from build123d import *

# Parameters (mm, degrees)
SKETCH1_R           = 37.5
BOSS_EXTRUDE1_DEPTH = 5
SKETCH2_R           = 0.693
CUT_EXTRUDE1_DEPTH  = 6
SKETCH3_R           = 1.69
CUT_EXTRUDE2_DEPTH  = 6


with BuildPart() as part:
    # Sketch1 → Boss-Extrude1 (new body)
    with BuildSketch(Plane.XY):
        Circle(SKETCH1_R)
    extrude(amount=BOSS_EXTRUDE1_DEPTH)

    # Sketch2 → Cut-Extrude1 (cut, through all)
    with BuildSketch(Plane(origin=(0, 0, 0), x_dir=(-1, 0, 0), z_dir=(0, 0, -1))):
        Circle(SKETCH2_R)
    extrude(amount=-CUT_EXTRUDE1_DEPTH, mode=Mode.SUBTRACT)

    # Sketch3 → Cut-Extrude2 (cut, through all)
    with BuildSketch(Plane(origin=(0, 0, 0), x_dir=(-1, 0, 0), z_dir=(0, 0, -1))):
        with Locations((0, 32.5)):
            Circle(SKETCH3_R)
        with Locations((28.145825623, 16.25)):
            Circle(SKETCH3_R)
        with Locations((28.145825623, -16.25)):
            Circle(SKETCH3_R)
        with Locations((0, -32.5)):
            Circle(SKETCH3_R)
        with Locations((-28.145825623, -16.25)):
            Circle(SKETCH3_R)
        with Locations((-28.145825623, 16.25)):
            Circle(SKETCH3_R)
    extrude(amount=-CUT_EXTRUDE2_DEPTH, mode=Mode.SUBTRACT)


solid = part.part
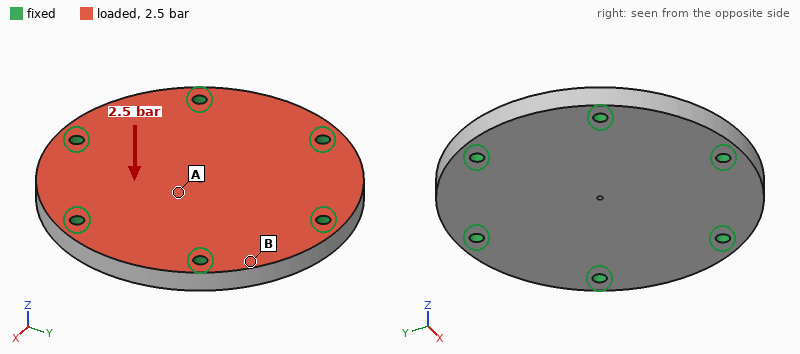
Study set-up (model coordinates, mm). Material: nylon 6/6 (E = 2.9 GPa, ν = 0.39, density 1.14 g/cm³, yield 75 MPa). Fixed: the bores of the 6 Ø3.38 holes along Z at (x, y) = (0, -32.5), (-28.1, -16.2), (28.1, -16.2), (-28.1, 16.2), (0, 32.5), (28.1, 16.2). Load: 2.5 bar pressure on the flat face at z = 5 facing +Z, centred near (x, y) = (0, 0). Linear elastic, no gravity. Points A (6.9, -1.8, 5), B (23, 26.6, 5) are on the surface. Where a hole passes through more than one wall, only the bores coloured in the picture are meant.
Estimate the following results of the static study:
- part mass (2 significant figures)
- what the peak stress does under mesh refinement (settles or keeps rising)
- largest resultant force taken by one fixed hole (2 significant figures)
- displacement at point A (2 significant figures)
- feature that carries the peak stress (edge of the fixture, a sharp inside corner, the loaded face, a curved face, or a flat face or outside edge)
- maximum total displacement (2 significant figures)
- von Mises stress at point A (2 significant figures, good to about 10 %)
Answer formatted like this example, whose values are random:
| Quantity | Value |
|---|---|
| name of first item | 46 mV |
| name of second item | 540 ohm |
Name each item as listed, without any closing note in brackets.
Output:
| Quantity | Value |
|---|---|
| part mass | 25 g |
| what the peak stress does under mesh refinement | keeps rising |
| largest resultant force taken by one fixed hole | 180 N |
| displacement at point A | 0.18 mm |
| feature that carries the peak stress | edge of the fixture |
| maximum total displacement | 0.20 mm |
| von Mises stress at point A | 5.7 MPa |
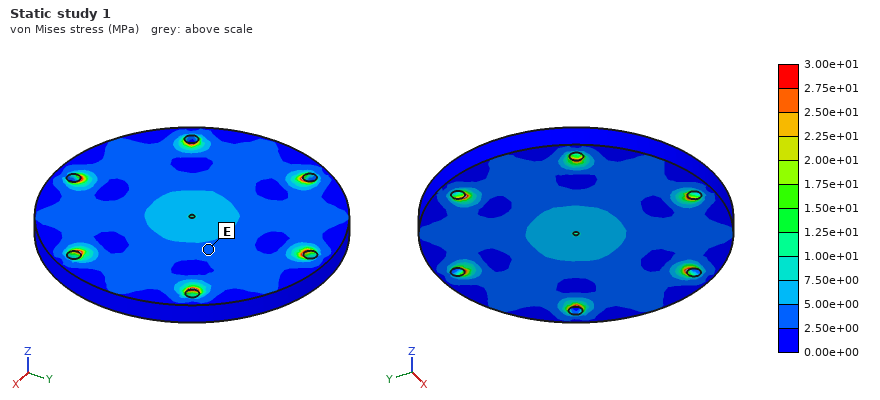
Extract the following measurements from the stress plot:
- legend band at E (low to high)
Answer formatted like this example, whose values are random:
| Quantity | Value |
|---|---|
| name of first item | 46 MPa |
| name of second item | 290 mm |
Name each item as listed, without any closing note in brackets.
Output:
| Quantity | Value |
|---|---|
| legend band at E | 2.50e+00 to 5.00e+00 MPa |
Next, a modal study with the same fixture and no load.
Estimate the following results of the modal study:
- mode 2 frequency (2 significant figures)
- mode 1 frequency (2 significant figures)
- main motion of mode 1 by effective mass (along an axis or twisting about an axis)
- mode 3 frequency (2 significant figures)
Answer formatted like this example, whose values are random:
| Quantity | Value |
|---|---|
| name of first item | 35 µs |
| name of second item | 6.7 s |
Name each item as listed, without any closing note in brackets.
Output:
| Quantity | Value |
|---|---|
| mode 2 frequency | 5700 Hz |
| mode 1 frequency | 2900 Hz |
| main motion of mode 1 by effective mass | along Z |
| mode 3 frequency | 5700 Hz |
